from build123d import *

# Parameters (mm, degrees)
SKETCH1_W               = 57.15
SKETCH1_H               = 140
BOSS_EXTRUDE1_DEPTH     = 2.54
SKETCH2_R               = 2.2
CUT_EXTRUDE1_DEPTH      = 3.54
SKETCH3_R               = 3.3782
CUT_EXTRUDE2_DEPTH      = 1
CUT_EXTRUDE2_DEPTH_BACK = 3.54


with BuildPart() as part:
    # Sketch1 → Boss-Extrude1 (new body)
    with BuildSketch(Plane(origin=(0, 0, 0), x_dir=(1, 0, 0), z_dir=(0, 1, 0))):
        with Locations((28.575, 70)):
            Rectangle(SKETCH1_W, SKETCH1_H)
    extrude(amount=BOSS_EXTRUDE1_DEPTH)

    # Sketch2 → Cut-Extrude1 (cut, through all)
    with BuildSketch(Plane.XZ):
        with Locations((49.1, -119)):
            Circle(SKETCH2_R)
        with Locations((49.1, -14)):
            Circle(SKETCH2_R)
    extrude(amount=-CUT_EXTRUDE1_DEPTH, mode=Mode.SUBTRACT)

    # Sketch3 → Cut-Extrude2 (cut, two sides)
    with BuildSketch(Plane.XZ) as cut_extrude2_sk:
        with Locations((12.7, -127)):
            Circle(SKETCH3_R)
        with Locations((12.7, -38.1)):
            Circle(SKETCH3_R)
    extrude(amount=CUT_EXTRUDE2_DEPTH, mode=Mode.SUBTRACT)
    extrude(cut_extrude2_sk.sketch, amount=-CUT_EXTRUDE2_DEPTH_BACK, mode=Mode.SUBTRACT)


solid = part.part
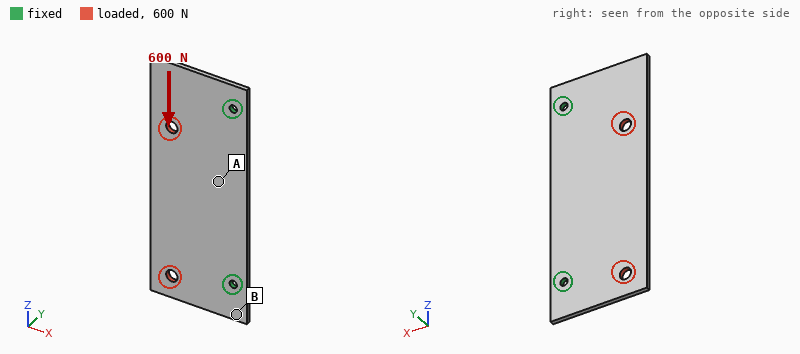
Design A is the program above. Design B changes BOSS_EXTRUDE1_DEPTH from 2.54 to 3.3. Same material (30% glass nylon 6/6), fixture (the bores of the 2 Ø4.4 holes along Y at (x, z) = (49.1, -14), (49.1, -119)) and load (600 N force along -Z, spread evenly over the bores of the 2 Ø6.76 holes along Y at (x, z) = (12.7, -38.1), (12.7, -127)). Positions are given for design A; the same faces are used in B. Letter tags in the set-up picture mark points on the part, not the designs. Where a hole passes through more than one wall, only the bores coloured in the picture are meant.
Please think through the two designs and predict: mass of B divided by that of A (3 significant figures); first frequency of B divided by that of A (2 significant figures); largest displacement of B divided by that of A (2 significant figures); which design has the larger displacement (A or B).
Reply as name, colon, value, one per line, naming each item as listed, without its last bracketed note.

mass of B divided by that of A: 1.30
first frequency of B divided by that of A: 1.3
largest displacement of B divided by that of A: 0.77
which design has the larger displacement: A
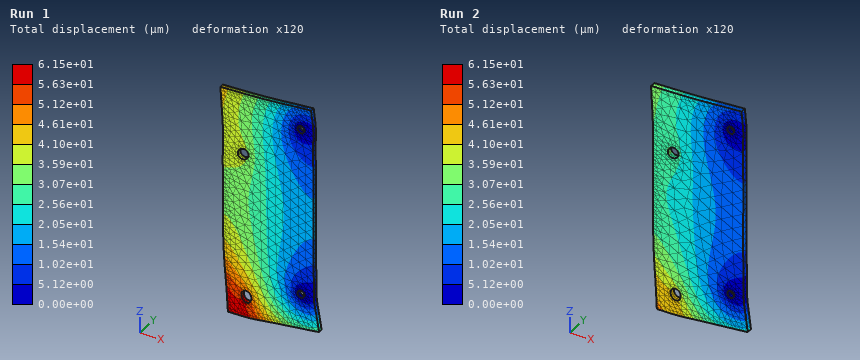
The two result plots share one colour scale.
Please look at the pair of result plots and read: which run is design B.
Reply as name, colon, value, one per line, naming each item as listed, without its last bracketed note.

which run is design B: Run 2
